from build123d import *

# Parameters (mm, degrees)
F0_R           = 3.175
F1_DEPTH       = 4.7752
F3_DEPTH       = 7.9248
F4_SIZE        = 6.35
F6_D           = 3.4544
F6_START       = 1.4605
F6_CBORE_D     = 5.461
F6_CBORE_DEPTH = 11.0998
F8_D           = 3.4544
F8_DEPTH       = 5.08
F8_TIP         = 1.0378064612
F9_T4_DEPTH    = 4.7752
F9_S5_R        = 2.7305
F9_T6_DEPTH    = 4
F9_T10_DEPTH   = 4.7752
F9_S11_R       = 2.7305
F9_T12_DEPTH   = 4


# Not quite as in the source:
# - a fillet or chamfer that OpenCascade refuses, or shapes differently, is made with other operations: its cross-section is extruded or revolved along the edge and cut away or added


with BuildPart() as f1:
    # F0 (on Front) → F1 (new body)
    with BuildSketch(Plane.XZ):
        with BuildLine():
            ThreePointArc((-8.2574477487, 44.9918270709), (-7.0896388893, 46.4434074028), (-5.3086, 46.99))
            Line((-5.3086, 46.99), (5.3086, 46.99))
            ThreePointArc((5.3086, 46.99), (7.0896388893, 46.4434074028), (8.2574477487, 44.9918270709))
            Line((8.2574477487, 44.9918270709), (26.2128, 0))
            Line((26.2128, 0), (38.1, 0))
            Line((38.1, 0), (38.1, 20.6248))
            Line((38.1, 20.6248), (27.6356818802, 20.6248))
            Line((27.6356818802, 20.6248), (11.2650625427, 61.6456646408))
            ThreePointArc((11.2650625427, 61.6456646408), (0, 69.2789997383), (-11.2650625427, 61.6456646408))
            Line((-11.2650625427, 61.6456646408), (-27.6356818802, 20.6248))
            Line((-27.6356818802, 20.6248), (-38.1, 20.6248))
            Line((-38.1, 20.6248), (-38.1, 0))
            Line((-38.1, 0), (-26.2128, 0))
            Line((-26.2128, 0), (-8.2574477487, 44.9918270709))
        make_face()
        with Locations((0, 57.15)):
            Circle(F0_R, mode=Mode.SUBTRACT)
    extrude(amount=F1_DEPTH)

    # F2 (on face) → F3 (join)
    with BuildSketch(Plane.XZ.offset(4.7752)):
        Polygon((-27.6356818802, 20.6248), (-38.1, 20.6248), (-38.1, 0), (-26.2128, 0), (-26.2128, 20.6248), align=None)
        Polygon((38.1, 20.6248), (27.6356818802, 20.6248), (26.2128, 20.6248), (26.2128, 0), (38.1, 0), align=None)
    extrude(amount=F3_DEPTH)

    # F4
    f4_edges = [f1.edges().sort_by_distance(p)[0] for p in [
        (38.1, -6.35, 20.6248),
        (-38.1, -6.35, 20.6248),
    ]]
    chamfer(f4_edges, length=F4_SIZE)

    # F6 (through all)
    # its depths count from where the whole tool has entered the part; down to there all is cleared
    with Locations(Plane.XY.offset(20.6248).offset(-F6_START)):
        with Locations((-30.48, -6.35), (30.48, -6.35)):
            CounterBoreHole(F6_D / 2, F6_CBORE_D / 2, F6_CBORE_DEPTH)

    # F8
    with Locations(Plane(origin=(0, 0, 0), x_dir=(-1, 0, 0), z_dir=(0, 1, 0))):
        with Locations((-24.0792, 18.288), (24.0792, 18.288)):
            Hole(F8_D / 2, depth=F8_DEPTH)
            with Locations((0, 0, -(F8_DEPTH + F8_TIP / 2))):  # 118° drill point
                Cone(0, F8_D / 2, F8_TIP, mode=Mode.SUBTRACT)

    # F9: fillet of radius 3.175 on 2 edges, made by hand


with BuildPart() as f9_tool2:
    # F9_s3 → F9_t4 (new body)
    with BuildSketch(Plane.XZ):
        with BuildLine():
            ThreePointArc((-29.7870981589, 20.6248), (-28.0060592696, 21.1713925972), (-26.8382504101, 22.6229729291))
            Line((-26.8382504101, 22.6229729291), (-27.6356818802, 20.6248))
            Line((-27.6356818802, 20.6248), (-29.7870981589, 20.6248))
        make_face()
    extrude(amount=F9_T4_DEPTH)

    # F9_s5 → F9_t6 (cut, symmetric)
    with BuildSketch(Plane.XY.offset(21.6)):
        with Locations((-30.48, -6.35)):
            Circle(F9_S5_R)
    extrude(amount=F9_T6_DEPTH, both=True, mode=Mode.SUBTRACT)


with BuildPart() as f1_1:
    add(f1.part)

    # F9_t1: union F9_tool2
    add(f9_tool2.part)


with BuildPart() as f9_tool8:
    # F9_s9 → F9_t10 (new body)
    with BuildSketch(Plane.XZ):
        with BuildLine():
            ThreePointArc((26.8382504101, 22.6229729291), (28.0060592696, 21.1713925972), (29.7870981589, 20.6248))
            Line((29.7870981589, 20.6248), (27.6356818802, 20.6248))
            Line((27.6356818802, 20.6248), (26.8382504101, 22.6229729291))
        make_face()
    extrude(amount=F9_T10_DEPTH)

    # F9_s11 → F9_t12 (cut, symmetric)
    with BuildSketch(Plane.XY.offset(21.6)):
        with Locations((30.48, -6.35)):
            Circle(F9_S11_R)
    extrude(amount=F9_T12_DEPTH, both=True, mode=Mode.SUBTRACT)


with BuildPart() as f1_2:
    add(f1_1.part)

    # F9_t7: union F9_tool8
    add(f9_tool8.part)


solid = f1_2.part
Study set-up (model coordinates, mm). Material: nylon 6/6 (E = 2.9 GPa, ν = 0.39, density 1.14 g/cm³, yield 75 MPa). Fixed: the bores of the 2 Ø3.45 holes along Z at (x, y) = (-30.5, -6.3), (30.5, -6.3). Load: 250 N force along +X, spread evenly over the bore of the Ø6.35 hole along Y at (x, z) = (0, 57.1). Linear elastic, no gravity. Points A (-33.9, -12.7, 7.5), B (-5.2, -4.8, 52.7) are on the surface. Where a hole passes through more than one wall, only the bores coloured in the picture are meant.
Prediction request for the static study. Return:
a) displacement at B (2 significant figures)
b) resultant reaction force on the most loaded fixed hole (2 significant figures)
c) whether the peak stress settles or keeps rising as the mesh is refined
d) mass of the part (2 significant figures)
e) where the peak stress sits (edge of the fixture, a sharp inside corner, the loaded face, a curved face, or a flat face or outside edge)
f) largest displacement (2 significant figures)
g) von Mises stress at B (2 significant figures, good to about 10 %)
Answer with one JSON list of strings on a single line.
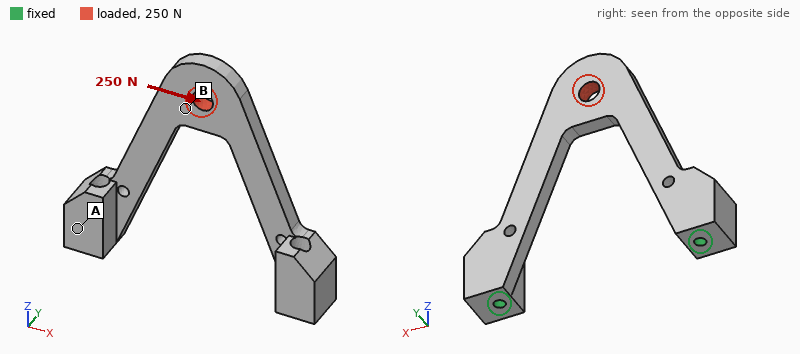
["0.37 mm", "220 N", "keeps rising", "12 g", "edge of the fixture", "0.40 mm", "6.2 MPa"]
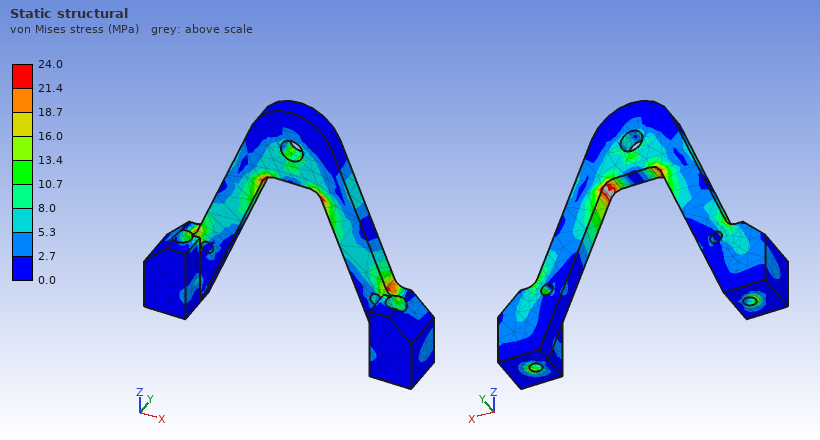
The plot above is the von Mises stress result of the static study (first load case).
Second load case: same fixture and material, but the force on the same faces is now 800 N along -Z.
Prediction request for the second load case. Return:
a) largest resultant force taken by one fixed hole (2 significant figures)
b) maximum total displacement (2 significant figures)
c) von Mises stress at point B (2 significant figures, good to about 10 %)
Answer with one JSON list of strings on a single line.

["440 N", "0.46 mm", "8.7 MPa"]
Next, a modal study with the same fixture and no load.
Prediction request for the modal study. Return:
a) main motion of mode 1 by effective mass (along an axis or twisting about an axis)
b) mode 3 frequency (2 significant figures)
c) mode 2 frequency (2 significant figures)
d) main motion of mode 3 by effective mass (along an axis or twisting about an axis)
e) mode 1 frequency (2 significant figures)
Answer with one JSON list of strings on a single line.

["along Y", "1900 Hz", "1500 Hz", "along X", "340 Hz"]
